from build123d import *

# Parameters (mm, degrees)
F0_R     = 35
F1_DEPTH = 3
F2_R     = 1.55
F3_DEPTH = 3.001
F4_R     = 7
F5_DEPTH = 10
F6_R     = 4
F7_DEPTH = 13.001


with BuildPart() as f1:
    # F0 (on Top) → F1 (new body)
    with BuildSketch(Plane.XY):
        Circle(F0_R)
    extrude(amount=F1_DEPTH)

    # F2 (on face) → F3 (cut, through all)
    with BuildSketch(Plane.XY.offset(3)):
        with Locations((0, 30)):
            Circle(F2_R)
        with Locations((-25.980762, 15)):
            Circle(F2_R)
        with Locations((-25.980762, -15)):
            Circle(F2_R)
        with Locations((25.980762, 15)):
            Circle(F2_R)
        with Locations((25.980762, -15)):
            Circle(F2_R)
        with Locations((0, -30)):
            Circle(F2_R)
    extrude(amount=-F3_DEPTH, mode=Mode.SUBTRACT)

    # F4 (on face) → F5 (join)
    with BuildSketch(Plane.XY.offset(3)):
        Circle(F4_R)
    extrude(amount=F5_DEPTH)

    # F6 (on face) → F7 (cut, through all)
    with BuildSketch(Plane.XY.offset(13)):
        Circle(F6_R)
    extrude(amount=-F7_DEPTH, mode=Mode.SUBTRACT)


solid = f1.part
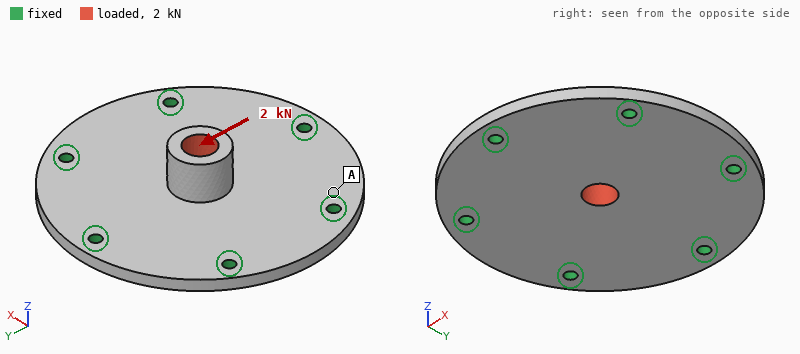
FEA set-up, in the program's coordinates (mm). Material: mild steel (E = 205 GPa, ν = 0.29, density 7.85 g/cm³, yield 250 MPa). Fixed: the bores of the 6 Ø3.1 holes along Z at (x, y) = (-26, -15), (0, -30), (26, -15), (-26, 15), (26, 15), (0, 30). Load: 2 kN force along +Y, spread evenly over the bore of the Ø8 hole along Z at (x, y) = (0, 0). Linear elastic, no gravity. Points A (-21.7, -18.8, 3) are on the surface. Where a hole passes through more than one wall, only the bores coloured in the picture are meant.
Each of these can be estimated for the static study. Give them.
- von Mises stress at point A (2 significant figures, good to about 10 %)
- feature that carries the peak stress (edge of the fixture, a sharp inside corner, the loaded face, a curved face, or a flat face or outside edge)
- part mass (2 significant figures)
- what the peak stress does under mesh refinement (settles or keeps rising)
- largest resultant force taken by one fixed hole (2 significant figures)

8.5 MPa
edge of the fixture
97 g
keeps rising
520 N
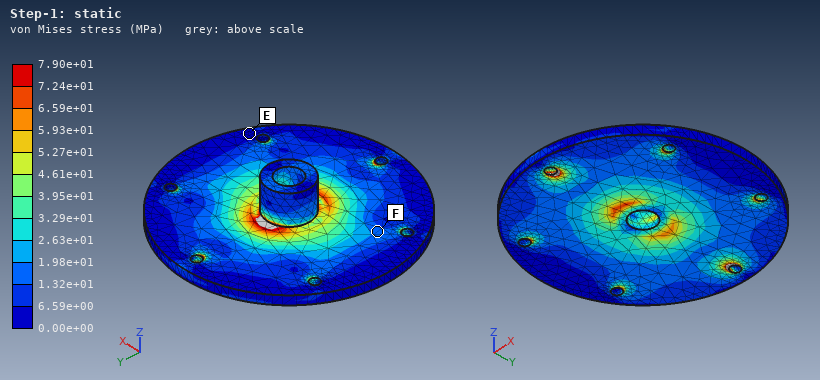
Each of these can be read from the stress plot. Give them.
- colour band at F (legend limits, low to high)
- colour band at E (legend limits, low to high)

1.32e+01 to 1.98e+01 MPa
0.00e+00 to 6.59e+00 MPa
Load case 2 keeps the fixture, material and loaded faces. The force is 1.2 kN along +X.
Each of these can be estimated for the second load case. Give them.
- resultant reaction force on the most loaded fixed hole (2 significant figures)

270 N
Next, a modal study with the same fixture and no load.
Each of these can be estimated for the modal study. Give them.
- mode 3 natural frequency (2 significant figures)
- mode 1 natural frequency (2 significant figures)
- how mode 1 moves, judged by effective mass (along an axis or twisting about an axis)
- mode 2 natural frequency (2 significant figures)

12 kHz
6100 Hz
along Z
12 kHz
